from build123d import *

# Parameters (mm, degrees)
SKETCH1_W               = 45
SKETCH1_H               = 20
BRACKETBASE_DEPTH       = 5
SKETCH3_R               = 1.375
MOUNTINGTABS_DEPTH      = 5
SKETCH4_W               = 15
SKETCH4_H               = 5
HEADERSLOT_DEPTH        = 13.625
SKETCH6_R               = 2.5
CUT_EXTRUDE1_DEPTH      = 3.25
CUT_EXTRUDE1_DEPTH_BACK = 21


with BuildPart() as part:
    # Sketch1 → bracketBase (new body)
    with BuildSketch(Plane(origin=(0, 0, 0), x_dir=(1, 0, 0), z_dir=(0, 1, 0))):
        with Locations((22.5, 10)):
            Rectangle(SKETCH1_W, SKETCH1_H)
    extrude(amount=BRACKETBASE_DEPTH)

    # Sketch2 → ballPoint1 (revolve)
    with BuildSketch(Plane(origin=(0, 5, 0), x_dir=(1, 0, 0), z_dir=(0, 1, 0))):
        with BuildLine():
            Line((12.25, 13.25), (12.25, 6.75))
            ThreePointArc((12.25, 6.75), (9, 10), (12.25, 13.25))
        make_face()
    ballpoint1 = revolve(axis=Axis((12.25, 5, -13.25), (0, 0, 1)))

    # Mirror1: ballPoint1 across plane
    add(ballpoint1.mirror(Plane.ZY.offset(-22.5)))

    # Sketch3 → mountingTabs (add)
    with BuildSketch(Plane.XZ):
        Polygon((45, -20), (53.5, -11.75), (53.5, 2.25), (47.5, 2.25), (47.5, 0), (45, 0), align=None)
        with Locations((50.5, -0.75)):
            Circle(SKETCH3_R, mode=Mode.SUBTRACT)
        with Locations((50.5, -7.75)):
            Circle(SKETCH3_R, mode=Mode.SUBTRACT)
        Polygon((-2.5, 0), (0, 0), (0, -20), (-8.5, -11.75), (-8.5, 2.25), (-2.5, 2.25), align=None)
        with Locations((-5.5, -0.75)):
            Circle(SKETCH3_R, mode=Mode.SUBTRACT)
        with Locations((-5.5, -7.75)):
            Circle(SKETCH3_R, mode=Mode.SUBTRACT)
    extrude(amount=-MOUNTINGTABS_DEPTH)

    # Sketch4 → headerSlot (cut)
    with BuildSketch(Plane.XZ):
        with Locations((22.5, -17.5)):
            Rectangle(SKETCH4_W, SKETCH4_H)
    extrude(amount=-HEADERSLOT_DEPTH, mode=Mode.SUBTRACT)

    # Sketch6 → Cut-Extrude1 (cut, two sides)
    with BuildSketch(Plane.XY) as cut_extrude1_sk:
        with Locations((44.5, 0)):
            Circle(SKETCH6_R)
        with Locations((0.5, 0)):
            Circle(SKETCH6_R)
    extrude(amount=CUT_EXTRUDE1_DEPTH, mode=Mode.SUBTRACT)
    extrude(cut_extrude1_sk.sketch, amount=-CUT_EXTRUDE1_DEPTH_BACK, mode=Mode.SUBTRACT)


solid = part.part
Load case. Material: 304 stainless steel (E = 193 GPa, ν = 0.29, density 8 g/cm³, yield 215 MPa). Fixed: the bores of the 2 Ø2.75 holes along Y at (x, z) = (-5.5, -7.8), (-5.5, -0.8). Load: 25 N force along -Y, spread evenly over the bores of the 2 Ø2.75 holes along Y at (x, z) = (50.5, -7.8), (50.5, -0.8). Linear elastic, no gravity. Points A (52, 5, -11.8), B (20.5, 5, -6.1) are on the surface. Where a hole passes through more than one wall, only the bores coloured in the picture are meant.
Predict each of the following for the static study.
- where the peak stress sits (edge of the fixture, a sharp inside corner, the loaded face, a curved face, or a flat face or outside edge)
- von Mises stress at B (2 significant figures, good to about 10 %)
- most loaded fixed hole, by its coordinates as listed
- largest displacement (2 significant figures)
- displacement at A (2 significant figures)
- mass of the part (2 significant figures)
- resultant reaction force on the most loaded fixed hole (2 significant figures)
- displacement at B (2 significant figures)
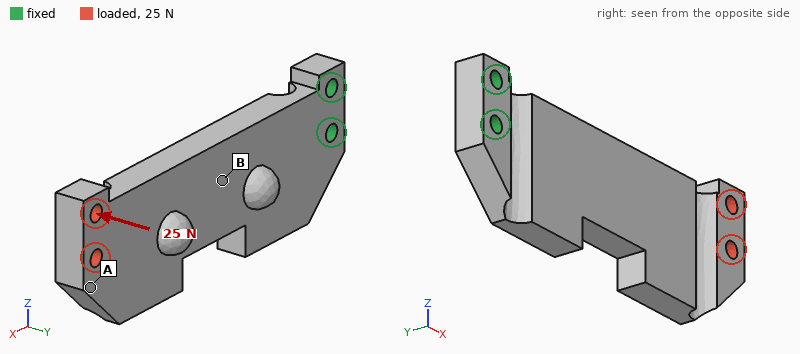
a curved face
12 MPa
(-5.5, -7.8)
98 µm
93 µm
42 g
19 N
31 µm
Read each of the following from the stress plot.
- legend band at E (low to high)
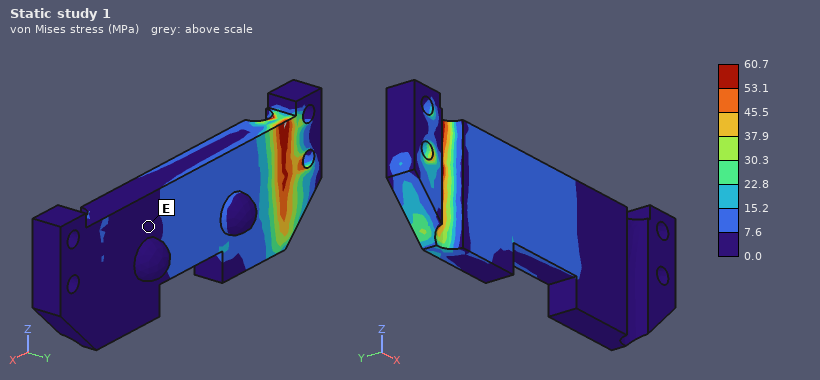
0.0 to 7.6 MPa
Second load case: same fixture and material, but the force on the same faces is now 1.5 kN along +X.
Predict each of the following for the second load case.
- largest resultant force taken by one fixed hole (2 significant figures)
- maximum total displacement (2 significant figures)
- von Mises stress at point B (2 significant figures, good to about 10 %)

800 N
0.11 mm
25 MPa
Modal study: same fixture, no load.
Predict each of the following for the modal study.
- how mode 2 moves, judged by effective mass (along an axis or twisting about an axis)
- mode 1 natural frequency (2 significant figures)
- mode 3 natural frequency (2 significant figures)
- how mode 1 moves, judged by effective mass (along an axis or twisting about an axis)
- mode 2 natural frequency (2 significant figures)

along Z
760 Hz
5300 Hz
along Y
2600 Hz
